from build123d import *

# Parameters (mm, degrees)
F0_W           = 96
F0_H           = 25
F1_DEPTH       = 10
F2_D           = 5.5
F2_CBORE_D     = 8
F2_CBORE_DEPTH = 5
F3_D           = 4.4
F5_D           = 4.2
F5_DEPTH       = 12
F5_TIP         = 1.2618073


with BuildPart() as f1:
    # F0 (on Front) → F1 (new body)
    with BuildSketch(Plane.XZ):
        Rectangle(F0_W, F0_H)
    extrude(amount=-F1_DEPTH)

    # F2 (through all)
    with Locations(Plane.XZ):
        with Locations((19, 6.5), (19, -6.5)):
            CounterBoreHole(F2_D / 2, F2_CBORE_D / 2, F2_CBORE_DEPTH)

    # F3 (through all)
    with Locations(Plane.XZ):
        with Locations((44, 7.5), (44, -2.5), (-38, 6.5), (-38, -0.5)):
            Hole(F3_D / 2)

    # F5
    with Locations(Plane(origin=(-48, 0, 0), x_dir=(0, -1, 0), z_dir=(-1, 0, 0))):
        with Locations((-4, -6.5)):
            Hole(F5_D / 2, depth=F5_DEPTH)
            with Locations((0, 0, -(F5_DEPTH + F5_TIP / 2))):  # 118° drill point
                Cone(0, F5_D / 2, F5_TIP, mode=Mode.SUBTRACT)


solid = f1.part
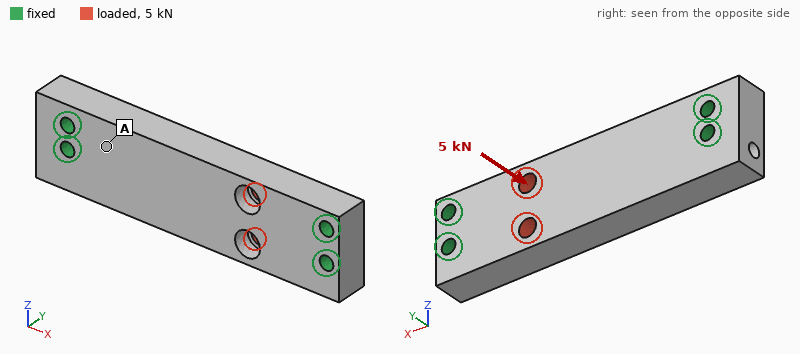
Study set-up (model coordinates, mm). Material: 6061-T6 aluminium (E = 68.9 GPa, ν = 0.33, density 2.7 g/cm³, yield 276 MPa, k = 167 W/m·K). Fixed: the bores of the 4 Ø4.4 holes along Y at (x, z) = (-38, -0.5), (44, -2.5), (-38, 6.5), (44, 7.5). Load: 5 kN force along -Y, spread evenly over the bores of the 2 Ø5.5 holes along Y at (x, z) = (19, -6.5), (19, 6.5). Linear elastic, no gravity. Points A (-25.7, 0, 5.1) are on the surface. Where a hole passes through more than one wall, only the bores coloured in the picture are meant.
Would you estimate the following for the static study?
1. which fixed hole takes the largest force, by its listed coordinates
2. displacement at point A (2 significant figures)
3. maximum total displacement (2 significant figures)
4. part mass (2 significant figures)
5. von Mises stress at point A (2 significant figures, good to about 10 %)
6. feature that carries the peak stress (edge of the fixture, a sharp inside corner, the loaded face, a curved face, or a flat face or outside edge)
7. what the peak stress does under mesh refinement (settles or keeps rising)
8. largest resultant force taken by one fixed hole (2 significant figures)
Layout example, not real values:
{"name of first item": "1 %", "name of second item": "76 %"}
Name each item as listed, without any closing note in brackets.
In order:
{"which fixed hole takes the largest force, by its listed coordinates": "(44, -2.5)", "displacement at point A": "16 µm", "maximum total displacement": "98 µm", "part mass": "61 g", "von Mises stress at point A": "37 MPa", "feature that carries the peak stress": "edge of the fixture", "what the peak stress does under mesh refinement": "keeps rising", "largest resultant force taken by one fixed hole": "2.4 kN"}
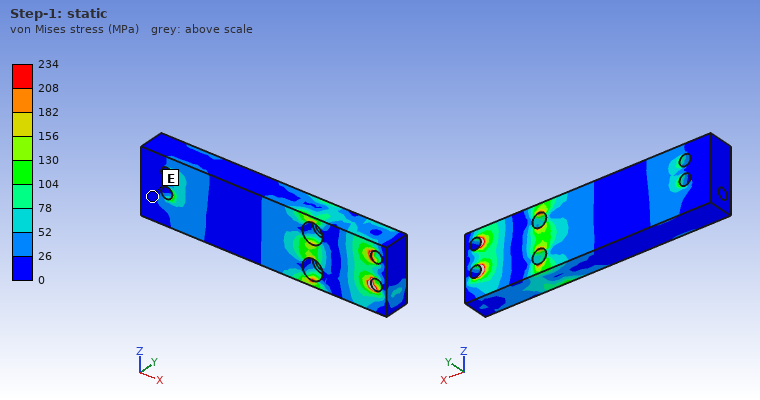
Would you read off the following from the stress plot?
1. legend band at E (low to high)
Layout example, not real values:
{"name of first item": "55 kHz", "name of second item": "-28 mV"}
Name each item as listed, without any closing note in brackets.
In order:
{"legend band at E": "0 to 26 MPa"}
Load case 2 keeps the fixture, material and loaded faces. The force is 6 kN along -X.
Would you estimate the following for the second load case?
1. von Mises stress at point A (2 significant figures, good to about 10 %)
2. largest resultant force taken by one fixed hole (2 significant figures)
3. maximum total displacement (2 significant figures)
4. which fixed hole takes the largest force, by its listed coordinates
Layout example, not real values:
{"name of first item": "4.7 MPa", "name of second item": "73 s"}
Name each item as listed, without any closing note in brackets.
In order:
{"von Mises stress at point A": "14 MPa", "largest resultant force taken by one fixed hole": "2.4 kN", "maximum total displacement": "12 µm", "which fixed hole takes the largest force, by its listed coordinates": "(44, -2.5)"}
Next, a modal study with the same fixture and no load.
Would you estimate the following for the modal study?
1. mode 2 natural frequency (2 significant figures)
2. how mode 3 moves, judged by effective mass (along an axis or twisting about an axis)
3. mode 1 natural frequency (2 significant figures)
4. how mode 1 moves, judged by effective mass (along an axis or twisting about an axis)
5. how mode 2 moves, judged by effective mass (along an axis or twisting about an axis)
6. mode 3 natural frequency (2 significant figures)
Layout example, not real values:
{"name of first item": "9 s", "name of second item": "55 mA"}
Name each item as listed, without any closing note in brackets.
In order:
{"mode 2 natural frequency": "11 kHz", "how mode 3 moves, judged by effective mass": "twisting about X", "mode 1 natural frequency": "7100 Hz", "how mode 1 moves, judged by effective mass": "along Y", "how mode 2 moves, judged by effective mass": "along Z", "mode 3 natural frequency": "13 kHz"}
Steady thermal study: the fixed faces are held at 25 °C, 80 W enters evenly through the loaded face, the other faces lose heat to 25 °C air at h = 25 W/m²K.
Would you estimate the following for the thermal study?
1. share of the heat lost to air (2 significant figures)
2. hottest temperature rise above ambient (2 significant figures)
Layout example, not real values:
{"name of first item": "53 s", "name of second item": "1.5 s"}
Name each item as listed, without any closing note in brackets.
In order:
{"share of the heat lost to air": "3.1 %", "hottest temperature rise above ambient": "38 K"}
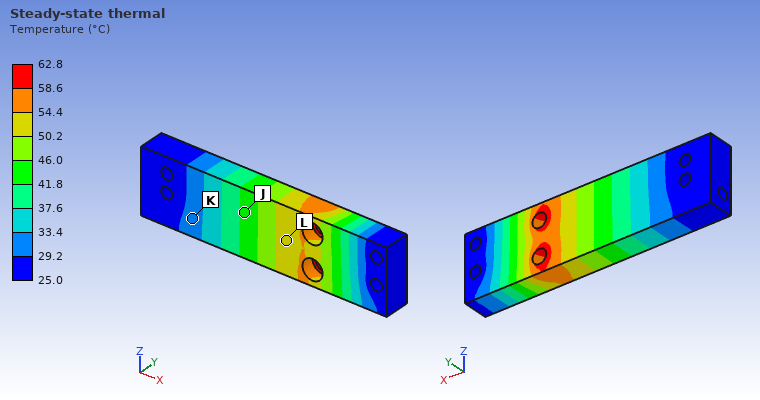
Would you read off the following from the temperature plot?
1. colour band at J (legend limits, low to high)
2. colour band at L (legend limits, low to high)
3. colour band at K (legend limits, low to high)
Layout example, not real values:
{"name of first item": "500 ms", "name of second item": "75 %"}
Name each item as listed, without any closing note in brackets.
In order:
{"colour band at J": "41.8 to 46.0 °C", "colour band at L": "50.2 to 54.4 °C", "colour band at K": "29.2 to 33.4 °C"}
